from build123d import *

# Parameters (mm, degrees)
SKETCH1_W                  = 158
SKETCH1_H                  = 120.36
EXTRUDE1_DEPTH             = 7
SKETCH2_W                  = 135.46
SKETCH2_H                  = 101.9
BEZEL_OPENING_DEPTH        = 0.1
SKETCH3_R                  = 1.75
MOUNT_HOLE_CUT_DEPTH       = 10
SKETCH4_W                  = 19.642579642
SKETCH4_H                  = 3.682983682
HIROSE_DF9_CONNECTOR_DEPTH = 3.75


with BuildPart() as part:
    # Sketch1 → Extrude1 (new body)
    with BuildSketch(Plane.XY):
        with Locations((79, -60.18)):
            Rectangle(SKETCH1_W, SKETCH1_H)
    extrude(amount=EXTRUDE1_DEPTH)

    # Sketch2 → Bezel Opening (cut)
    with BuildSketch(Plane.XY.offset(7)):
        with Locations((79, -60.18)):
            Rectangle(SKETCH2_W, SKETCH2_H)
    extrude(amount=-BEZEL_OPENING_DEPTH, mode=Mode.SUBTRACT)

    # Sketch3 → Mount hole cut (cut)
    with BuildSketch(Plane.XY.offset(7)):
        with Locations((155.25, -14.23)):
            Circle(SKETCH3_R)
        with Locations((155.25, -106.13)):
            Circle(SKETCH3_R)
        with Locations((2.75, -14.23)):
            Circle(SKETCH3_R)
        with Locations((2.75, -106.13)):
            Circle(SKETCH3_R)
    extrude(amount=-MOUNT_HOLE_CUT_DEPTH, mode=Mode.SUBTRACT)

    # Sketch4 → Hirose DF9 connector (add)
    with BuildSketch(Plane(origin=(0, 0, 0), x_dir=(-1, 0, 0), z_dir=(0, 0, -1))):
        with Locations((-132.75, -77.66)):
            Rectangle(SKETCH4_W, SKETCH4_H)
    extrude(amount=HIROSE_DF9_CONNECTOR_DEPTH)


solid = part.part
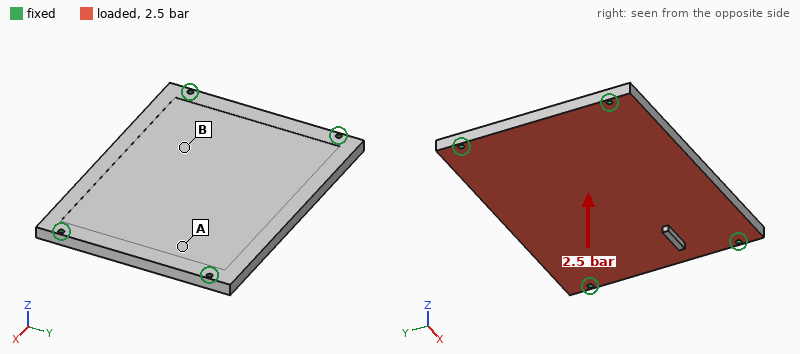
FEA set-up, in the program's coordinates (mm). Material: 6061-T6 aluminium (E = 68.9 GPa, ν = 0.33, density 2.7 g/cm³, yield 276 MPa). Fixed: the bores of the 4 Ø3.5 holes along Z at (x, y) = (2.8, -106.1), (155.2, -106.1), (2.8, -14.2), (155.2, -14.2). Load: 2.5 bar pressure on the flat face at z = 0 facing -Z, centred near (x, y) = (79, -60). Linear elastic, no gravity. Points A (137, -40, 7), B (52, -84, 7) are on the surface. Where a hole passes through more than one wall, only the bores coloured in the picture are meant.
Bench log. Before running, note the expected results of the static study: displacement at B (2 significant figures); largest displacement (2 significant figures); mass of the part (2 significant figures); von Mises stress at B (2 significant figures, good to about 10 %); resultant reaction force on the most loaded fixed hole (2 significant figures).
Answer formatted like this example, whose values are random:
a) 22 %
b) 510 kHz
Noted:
a) 0.28 mm
b) 0.34 mm
c) 360 g
d) 29 MPa
e) 1.2 kN
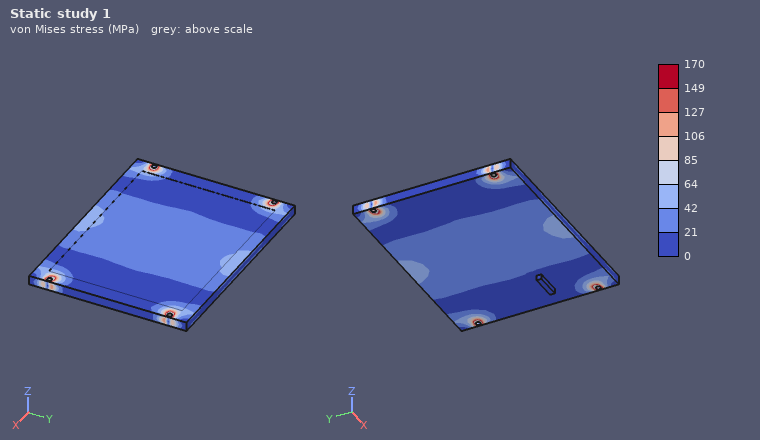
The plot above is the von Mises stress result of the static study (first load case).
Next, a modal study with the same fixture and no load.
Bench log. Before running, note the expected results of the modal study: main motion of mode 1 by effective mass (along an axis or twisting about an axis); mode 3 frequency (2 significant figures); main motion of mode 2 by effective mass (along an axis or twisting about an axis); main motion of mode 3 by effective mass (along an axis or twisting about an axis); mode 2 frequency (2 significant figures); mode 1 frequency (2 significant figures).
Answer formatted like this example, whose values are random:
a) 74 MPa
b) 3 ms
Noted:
a) along Z
b) 3000 Hz
c) twisting about X
d) twisting about Y
e) 1800 Hz
f) 1100 Hz
